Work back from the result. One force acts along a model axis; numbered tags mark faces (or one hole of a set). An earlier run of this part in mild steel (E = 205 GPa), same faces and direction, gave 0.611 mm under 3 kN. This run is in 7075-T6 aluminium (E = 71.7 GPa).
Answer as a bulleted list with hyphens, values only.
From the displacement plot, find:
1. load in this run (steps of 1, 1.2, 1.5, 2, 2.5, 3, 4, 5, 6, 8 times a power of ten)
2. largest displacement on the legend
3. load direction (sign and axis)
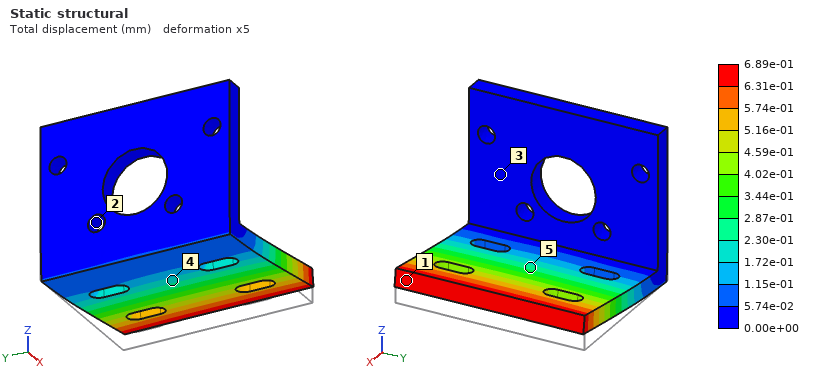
- 1.2 kN
- 6.89e-01 mm
- +Z
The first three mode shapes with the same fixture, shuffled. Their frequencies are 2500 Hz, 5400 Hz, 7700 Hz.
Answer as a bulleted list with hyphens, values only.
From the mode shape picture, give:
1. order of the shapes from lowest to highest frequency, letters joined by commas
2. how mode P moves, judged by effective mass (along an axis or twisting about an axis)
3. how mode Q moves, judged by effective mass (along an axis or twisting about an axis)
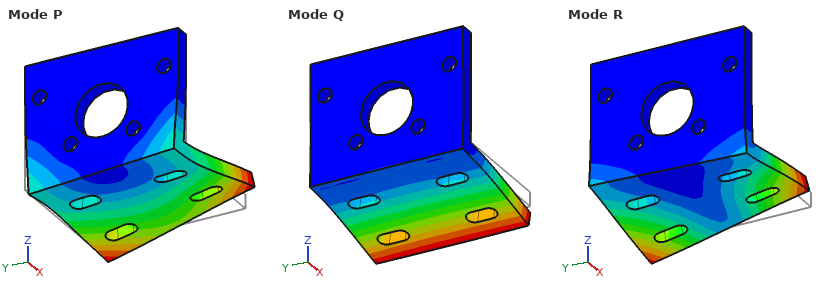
- Q, R, P
- along Y
- along Z
